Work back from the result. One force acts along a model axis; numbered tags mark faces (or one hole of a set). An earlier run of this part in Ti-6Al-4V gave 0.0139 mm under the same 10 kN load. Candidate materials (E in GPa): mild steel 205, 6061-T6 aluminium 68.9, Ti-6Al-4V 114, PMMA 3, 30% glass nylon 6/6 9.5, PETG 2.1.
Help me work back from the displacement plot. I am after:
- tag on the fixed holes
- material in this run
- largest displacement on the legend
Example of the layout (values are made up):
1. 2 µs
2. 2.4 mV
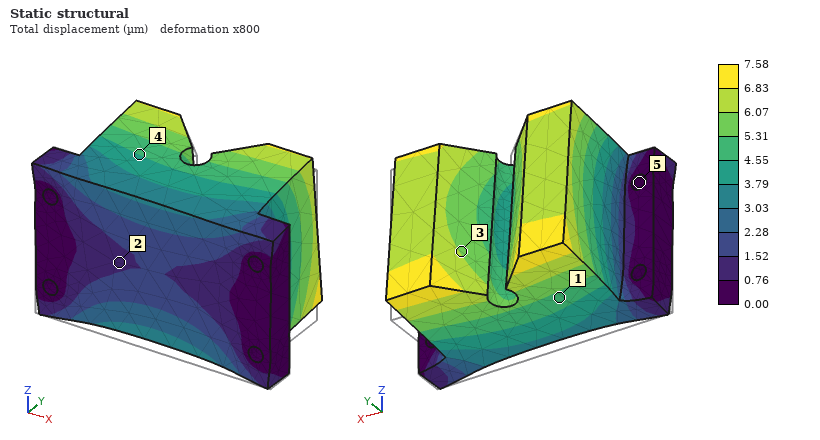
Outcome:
1. 5
2. mild steel
3. 7.58 µm
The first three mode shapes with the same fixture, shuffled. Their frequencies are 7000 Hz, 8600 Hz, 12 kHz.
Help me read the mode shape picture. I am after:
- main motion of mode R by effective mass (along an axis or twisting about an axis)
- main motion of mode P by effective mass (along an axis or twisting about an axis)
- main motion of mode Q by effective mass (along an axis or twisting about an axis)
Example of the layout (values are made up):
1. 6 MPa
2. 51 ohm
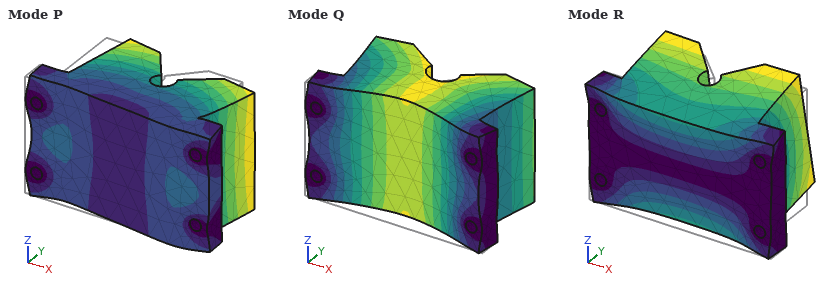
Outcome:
1. along Z
2. along X
3. along Y
